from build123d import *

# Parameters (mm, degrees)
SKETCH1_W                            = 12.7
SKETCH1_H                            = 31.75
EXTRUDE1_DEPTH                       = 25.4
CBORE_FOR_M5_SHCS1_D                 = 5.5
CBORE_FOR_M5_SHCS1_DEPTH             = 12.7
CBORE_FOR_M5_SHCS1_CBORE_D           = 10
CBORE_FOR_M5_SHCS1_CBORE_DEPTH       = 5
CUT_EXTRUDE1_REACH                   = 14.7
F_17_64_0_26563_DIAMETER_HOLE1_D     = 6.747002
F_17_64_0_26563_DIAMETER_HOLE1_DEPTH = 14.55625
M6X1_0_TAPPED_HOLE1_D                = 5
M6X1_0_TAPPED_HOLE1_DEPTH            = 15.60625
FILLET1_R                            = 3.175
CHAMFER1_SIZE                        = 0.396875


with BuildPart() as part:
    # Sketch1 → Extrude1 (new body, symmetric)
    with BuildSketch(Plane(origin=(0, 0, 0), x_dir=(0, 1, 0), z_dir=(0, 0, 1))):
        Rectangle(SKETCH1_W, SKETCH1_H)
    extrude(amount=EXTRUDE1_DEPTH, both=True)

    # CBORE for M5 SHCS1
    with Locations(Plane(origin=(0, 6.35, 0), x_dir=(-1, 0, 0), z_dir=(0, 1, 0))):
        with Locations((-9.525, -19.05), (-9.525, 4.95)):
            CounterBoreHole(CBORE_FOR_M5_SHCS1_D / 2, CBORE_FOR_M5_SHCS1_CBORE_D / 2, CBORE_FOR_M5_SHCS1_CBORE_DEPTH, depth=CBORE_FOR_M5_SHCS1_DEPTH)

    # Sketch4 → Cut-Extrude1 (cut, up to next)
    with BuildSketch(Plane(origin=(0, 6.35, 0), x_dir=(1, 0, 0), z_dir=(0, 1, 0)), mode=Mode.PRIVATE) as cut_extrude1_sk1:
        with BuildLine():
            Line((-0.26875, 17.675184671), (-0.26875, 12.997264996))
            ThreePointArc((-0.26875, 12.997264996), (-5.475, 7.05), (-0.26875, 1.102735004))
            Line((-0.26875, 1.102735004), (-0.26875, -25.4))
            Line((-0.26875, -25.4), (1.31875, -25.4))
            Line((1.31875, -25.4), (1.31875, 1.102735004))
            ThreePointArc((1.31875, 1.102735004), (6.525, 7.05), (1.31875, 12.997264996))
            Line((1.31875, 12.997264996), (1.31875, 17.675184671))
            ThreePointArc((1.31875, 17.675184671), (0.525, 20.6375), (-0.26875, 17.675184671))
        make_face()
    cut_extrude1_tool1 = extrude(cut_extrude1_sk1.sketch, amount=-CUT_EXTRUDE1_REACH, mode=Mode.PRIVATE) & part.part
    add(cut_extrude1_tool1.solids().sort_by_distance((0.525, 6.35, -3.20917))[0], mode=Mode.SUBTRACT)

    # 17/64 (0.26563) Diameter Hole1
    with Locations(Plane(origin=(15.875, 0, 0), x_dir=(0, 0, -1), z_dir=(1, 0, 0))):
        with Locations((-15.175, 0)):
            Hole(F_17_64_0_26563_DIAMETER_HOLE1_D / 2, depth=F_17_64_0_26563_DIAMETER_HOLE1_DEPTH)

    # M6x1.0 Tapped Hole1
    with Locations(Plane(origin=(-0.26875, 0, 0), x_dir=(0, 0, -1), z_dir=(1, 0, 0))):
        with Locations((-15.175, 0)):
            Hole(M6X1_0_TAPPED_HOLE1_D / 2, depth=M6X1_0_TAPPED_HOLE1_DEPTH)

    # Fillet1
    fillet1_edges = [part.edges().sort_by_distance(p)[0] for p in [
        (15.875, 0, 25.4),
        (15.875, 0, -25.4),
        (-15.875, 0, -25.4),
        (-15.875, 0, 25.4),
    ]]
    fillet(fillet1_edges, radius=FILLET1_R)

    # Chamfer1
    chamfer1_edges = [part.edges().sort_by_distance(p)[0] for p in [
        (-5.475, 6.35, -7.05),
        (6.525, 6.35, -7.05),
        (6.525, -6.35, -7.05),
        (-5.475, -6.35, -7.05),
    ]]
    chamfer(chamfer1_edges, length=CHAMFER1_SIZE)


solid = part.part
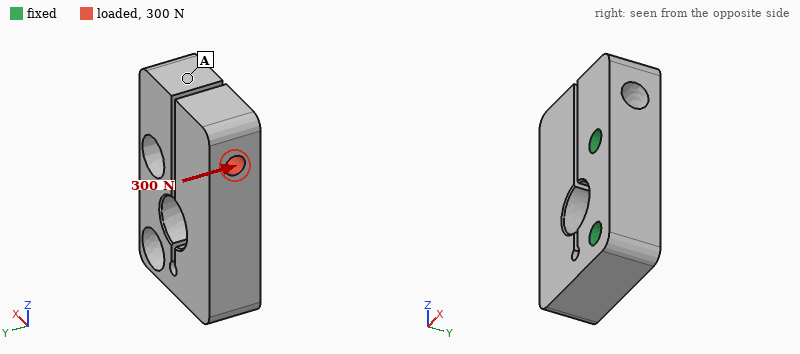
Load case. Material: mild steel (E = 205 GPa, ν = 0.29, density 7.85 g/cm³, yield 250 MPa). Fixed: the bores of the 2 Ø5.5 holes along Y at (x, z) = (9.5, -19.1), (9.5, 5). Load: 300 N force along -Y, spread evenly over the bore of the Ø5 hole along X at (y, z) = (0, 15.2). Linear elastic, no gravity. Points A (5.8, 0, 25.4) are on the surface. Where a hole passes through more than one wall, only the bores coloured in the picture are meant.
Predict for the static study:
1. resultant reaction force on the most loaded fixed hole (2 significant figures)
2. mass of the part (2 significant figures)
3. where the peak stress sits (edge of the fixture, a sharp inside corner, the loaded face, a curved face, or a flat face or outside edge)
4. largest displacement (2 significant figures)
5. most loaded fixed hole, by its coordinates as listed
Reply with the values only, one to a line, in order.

230 N
130 g
a curved face
0.11 mm
(9.5, 5)
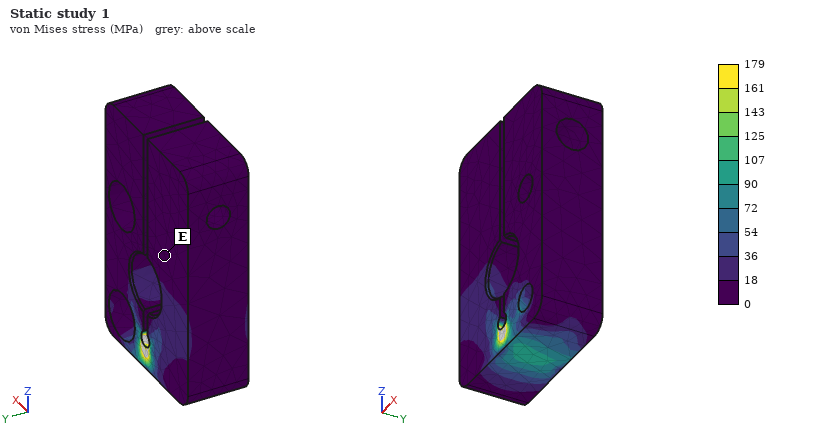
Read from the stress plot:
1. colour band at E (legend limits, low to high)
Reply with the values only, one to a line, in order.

0 to 18 MPa
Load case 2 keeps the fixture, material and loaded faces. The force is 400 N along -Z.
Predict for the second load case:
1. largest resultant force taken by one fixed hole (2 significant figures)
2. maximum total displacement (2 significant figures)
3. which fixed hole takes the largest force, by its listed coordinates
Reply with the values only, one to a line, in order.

360 N
57 µm
(9.5, -19.1)
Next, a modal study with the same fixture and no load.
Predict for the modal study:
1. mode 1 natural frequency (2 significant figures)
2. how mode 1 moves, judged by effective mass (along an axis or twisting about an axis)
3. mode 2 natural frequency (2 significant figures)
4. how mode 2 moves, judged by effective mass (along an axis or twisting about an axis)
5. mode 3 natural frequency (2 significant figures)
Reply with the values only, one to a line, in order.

1100 Hz
along X
1600 Hz
along Y
6100 Hz
